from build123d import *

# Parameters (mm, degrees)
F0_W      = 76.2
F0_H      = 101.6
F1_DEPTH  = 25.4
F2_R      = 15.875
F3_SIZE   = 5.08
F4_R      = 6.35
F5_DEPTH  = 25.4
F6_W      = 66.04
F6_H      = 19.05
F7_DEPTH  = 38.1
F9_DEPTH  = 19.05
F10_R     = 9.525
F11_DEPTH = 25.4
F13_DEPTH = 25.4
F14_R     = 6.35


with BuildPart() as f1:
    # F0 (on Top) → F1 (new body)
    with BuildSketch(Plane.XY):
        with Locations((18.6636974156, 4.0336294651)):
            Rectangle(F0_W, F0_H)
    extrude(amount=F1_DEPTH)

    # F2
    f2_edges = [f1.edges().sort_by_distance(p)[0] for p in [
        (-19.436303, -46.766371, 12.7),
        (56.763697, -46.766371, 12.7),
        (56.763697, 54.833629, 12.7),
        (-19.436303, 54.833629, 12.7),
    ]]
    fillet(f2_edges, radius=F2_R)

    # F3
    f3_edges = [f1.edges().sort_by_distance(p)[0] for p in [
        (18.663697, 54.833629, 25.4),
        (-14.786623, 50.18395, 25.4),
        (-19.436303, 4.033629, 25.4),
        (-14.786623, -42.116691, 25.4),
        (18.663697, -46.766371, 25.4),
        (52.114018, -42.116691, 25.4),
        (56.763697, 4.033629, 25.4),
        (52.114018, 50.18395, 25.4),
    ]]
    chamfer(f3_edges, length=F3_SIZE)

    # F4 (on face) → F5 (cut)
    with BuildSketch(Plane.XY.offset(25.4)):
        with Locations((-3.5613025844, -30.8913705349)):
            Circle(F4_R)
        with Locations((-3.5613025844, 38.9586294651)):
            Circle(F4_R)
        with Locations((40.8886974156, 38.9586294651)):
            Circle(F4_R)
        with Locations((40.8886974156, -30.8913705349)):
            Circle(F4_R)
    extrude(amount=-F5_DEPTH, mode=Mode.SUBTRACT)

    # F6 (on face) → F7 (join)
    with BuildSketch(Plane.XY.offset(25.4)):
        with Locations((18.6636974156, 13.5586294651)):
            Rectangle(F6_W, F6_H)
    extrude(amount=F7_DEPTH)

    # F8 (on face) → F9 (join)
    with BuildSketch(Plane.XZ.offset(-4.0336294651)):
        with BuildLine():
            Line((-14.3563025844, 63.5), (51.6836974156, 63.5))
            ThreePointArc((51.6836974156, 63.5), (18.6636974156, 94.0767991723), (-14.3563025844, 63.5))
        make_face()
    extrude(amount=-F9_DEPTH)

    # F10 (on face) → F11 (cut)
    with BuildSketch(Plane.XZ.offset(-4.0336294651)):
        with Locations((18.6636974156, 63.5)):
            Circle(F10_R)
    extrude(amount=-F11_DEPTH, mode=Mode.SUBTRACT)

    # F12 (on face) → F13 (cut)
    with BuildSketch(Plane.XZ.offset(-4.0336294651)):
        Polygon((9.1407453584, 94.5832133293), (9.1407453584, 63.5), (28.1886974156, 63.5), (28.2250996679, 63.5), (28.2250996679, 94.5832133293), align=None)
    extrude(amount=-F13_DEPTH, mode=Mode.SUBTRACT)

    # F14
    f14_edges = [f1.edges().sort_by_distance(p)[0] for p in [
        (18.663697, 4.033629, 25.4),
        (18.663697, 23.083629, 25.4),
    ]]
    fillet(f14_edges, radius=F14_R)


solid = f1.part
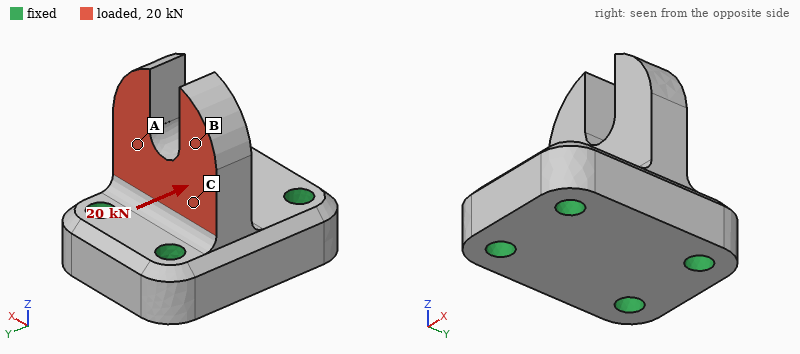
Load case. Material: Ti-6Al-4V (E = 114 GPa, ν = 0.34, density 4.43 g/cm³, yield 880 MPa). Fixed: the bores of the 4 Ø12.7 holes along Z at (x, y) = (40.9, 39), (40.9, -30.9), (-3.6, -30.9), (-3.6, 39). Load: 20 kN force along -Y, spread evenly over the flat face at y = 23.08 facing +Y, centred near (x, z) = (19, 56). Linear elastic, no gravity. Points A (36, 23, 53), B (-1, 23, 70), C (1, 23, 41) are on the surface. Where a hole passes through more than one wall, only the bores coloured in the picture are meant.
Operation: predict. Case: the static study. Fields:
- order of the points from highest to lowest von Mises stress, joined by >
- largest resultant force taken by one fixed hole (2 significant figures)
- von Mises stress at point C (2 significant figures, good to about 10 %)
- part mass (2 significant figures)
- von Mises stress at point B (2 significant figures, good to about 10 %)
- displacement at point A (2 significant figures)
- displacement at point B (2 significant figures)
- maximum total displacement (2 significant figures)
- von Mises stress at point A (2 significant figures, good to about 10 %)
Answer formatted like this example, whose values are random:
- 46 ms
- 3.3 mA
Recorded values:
- C > A > B
- 9.8 kN
- 82 MPa
- 1.1 kg
- 20 MPa
- 0.069 mm
- 0.12 mm
- 0.20 mm
- 55 MPa
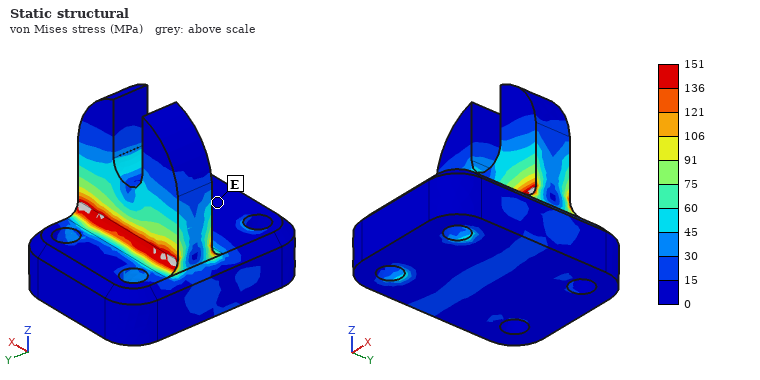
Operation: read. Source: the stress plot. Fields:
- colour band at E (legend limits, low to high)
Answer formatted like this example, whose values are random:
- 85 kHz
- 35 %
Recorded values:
- 0 to 15 MPa
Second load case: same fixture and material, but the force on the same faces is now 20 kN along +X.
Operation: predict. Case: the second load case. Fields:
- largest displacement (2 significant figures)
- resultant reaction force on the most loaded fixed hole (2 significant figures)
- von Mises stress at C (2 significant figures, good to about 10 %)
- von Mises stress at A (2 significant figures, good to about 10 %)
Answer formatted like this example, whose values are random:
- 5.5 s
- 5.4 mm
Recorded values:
- 91 µm
- 12 kN
- 48 MPa
- 48 MPa
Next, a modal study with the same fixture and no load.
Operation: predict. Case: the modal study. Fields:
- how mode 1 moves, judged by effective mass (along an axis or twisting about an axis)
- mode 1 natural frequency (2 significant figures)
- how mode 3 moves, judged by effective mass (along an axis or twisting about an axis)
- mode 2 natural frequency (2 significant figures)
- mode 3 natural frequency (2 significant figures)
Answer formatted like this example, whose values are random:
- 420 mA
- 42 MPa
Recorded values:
- along Y
- 4200 Hz
- along X
- 5500 Hz
- 6500 Hz
